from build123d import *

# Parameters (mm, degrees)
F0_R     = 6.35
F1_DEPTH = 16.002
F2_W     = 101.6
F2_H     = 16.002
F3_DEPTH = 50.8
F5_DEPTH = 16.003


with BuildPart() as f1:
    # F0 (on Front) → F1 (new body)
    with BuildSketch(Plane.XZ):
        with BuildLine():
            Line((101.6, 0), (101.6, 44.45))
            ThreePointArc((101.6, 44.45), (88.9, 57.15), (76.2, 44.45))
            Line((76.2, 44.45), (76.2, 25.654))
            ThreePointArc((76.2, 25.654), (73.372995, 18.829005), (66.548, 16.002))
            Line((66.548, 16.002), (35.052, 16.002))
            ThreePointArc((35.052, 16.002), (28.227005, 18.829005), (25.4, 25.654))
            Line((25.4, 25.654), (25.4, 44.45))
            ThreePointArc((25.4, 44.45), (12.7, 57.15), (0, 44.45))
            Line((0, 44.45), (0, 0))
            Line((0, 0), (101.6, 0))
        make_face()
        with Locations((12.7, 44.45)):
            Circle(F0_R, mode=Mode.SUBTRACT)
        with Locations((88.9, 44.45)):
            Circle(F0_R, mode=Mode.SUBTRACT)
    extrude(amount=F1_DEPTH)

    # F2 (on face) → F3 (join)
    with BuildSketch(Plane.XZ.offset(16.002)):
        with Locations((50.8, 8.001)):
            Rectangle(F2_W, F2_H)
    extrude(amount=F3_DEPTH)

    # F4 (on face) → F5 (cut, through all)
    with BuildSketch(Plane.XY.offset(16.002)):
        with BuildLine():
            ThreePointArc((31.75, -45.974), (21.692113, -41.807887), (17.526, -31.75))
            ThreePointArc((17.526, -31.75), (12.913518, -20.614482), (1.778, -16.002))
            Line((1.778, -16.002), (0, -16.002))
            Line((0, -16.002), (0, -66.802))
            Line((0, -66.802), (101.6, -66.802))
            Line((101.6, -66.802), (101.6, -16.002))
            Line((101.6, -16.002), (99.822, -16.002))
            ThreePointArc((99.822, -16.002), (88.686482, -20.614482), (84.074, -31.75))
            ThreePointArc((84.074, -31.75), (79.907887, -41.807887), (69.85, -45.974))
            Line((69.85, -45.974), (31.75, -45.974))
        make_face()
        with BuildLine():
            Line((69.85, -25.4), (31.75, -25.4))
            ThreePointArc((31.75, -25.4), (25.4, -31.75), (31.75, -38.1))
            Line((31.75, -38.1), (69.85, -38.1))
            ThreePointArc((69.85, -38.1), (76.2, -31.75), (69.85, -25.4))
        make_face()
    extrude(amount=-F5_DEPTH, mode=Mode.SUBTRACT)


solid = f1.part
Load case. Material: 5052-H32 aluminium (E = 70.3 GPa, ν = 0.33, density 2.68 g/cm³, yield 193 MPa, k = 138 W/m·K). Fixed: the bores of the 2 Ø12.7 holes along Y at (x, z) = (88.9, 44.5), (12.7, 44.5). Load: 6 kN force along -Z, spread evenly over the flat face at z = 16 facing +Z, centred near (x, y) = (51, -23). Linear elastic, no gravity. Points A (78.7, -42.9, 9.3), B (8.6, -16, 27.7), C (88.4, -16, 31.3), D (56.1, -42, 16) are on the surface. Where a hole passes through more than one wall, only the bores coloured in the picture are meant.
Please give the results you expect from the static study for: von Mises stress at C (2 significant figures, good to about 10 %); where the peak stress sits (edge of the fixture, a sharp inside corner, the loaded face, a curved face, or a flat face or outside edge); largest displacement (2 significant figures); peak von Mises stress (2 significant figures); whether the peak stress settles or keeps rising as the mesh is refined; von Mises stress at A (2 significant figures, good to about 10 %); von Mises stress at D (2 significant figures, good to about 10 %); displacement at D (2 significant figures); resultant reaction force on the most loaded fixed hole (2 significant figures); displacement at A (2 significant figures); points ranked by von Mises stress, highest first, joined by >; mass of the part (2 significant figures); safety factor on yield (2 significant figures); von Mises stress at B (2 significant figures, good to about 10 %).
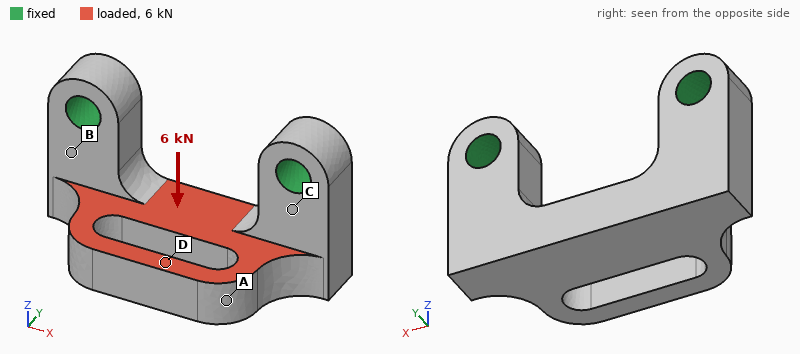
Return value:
57 MPa
a curved face
0.16 mm
92 MPa
settles
13 MPa
22 MPa
0.13 mm
3.3 kN
0.12 mm
C > B > D > A
200 g
2.1
45 MPa
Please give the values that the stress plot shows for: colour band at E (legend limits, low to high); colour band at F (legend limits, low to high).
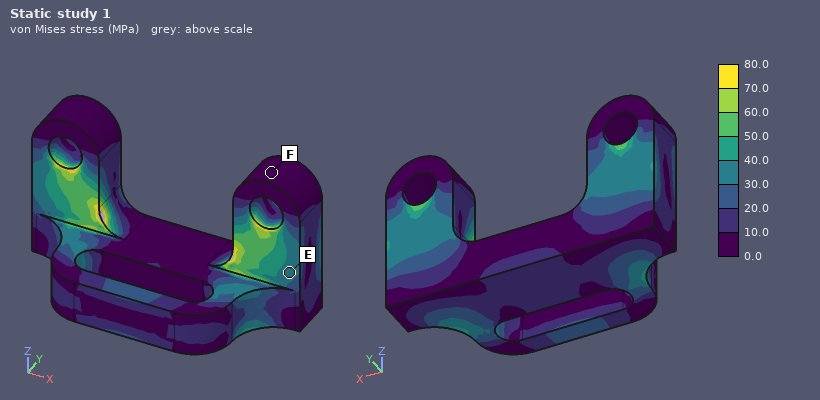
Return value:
30.0 to 40.0 MPa
0.0 to 10.0 MPa
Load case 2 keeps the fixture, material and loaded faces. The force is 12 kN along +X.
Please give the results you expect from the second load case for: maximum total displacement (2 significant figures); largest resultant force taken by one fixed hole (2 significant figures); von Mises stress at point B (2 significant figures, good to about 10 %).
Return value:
0.13 mm
6.4 kN
53 MPa
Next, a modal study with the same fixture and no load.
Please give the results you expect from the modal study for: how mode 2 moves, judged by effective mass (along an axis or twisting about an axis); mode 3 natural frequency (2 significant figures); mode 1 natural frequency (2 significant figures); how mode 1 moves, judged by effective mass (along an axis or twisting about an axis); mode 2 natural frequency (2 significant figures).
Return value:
along X
7000 Hz
3200 Hz
along Y
5700 Hz
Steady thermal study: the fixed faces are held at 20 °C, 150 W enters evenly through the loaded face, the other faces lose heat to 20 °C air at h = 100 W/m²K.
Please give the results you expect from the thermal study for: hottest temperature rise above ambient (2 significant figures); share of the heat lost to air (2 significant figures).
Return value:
61 K
28 %
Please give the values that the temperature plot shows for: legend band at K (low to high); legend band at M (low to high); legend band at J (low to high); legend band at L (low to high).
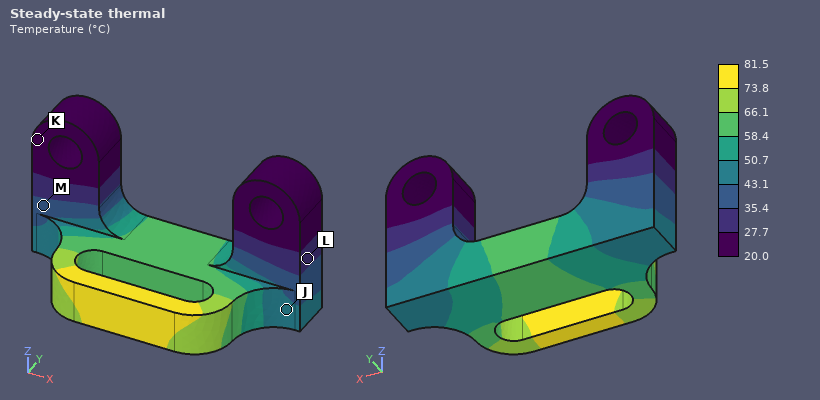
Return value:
20.0 to 27.7 °C
35.4 to 43.1 °C
43.1 to 50.7 °C
27.7 to 35.4 °C
